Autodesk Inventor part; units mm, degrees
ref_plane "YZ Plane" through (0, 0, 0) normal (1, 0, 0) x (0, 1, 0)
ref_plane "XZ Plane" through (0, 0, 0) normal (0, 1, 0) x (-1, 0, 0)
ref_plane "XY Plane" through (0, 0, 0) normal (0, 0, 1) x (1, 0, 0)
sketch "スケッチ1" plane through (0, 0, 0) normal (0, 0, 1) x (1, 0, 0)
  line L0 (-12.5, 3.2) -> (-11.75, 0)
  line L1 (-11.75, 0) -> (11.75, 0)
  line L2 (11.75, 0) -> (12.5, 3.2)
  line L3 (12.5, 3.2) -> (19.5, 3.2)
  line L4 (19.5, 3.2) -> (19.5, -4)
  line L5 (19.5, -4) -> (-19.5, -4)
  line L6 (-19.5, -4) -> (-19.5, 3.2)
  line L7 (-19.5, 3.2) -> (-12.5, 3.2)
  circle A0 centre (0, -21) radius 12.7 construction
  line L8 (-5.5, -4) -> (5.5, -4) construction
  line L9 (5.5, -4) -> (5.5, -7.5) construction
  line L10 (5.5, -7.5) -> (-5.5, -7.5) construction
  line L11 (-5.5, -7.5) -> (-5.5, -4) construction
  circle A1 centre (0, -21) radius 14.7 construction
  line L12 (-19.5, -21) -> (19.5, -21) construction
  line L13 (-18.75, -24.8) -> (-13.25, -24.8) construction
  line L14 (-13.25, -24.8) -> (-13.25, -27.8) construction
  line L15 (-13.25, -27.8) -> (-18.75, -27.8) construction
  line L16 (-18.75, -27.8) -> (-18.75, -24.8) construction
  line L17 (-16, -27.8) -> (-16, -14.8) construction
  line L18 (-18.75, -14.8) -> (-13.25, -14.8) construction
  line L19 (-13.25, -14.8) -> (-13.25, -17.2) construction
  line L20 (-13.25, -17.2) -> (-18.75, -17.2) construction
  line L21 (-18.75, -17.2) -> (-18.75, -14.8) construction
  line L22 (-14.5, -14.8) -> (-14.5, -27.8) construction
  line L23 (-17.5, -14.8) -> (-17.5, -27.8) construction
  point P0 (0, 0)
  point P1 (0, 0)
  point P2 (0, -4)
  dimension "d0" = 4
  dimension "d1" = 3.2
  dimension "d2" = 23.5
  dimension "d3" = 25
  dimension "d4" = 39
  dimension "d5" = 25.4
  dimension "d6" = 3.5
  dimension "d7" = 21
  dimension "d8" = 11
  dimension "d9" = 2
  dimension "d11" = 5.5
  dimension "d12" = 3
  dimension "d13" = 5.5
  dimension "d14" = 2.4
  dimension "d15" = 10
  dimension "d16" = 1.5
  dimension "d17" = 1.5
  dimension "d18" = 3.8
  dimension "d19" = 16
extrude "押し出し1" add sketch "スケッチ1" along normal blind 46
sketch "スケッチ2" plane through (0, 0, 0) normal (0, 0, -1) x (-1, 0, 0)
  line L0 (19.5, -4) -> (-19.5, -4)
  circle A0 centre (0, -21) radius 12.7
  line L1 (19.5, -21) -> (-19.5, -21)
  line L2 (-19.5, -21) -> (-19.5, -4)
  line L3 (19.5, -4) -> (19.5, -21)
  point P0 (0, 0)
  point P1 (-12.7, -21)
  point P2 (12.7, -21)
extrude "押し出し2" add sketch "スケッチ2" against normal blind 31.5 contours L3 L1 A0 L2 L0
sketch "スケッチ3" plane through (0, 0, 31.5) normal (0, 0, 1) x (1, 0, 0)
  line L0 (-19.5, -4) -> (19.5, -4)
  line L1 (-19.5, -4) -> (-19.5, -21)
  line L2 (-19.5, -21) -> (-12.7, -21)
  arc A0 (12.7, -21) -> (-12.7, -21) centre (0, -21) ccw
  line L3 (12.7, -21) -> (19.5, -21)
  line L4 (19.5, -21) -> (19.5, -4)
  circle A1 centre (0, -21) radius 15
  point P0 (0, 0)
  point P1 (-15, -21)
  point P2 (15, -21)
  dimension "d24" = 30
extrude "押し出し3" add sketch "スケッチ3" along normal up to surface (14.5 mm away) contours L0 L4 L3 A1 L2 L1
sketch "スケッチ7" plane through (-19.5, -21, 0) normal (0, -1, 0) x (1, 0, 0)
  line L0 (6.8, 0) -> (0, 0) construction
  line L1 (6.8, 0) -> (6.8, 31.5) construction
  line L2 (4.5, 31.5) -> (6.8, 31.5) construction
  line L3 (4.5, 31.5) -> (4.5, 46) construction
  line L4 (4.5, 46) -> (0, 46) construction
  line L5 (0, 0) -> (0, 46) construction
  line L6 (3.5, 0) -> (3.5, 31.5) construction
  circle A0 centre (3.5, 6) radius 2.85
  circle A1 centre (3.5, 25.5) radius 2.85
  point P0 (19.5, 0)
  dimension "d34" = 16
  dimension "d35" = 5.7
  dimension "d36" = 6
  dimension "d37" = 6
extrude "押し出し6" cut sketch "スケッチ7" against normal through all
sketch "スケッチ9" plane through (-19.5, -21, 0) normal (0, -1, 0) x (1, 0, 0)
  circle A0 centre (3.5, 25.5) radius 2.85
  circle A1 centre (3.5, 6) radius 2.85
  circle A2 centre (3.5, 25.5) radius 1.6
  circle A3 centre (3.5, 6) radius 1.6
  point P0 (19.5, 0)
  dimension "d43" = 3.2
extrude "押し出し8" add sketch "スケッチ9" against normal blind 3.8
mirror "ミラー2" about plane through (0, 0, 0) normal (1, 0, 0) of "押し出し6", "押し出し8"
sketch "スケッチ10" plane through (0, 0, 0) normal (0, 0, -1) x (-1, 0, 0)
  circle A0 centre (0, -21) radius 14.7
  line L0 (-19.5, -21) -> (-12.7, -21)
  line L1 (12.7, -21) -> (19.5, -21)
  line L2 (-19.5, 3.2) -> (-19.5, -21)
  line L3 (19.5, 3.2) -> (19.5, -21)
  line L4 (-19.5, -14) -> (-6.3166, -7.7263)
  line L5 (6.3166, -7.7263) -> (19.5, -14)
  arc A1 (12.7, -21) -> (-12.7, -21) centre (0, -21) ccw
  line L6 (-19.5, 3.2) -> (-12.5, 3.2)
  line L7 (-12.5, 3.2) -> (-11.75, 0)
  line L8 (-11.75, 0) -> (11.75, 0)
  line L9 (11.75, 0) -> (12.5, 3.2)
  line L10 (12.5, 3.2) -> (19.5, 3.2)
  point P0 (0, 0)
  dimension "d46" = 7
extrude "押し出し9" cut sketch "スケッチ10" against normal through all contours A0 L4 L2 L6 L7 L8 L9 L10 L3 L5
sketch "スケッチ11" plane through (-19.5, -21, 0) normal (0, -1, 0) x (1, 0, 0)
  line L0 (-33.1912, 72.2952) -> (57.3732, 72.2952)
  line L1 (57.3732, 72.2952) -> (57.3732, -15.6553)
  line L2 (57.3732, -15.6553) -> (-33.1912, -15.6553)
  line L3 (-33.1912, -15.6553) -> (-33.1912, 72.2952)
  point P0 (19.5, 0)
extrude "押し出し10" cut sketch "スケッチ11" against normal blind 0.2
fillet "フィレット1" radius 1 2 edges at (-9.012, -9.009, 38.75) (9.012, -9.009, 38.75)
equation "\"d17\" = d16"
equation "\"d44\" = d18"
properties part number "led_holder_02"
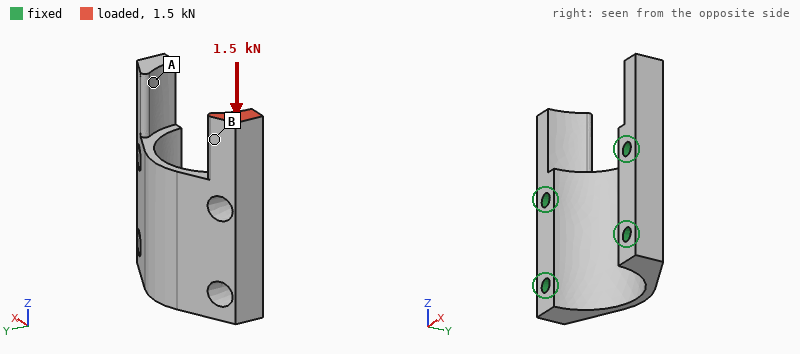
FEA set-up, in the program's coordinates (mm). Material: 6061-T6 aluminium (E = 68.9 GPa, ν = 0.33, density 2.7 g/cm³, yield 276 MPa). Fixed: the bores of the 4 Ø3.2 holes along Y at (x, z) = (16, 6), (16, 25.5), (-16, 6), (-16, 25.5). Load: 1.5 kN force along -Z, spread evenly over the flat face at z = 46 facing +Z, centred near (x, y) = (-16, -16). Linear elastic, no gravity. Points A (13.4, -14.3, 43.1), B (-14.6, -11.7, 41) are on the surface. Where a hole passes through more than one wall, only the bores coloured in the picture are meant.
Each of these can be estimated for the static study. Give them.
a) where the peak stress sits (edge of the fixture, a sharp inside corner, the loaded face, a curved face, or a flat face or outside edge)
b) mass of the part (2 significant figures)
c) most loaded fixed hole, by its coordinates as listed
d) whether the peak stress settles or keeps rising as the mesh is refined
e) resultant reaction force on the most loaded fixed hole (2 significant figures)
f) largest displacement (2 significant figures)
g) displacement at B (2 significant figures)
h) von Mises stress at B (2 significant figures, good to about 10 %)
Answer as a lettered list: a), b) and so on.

a) edge of the fixture
b) 18 g
c) (-16, 25.5)
d) keeps rising
e) 1.2 kN
f) 38 µm
g) 29 µm
h) 33 MPa
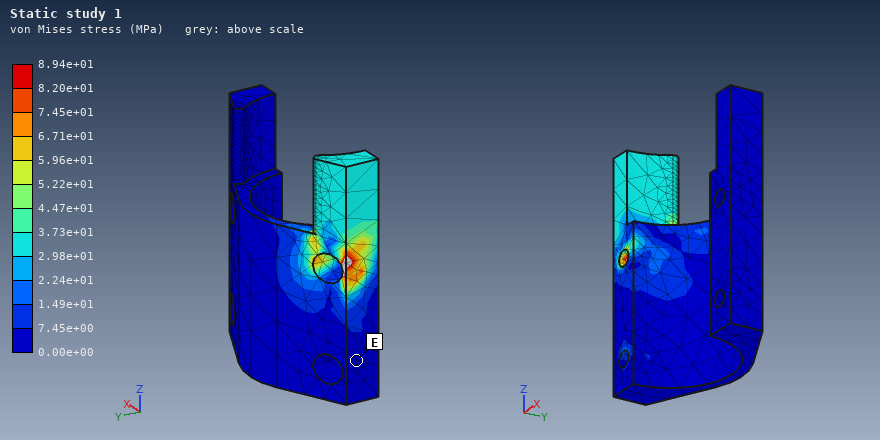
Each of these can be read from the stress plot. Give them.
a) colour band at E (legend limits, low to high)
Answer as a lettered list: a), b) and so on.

a) 0.00e+00 to 7.45e+00 MPa
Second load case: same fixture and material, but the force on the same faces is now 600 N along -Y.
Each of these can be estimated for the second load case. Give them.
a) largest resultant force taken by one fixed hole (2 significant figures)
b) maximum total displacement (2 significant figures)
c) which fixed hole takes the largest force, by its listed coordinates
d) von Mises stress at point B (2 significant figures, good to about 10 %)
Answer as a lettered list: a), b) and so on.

a) 1.1 kN
b) 0.18 mm
c) (-16, 25.5)
d) 46 MPa
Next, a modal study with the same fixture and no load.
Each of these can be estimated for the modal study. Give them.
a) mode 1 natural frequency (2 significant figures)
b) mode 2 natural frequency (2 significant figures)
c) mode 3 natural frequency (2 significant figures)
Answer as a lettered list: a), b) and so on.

a) 9600 Hz
b) 9700 Hz
c) 15 kHz
